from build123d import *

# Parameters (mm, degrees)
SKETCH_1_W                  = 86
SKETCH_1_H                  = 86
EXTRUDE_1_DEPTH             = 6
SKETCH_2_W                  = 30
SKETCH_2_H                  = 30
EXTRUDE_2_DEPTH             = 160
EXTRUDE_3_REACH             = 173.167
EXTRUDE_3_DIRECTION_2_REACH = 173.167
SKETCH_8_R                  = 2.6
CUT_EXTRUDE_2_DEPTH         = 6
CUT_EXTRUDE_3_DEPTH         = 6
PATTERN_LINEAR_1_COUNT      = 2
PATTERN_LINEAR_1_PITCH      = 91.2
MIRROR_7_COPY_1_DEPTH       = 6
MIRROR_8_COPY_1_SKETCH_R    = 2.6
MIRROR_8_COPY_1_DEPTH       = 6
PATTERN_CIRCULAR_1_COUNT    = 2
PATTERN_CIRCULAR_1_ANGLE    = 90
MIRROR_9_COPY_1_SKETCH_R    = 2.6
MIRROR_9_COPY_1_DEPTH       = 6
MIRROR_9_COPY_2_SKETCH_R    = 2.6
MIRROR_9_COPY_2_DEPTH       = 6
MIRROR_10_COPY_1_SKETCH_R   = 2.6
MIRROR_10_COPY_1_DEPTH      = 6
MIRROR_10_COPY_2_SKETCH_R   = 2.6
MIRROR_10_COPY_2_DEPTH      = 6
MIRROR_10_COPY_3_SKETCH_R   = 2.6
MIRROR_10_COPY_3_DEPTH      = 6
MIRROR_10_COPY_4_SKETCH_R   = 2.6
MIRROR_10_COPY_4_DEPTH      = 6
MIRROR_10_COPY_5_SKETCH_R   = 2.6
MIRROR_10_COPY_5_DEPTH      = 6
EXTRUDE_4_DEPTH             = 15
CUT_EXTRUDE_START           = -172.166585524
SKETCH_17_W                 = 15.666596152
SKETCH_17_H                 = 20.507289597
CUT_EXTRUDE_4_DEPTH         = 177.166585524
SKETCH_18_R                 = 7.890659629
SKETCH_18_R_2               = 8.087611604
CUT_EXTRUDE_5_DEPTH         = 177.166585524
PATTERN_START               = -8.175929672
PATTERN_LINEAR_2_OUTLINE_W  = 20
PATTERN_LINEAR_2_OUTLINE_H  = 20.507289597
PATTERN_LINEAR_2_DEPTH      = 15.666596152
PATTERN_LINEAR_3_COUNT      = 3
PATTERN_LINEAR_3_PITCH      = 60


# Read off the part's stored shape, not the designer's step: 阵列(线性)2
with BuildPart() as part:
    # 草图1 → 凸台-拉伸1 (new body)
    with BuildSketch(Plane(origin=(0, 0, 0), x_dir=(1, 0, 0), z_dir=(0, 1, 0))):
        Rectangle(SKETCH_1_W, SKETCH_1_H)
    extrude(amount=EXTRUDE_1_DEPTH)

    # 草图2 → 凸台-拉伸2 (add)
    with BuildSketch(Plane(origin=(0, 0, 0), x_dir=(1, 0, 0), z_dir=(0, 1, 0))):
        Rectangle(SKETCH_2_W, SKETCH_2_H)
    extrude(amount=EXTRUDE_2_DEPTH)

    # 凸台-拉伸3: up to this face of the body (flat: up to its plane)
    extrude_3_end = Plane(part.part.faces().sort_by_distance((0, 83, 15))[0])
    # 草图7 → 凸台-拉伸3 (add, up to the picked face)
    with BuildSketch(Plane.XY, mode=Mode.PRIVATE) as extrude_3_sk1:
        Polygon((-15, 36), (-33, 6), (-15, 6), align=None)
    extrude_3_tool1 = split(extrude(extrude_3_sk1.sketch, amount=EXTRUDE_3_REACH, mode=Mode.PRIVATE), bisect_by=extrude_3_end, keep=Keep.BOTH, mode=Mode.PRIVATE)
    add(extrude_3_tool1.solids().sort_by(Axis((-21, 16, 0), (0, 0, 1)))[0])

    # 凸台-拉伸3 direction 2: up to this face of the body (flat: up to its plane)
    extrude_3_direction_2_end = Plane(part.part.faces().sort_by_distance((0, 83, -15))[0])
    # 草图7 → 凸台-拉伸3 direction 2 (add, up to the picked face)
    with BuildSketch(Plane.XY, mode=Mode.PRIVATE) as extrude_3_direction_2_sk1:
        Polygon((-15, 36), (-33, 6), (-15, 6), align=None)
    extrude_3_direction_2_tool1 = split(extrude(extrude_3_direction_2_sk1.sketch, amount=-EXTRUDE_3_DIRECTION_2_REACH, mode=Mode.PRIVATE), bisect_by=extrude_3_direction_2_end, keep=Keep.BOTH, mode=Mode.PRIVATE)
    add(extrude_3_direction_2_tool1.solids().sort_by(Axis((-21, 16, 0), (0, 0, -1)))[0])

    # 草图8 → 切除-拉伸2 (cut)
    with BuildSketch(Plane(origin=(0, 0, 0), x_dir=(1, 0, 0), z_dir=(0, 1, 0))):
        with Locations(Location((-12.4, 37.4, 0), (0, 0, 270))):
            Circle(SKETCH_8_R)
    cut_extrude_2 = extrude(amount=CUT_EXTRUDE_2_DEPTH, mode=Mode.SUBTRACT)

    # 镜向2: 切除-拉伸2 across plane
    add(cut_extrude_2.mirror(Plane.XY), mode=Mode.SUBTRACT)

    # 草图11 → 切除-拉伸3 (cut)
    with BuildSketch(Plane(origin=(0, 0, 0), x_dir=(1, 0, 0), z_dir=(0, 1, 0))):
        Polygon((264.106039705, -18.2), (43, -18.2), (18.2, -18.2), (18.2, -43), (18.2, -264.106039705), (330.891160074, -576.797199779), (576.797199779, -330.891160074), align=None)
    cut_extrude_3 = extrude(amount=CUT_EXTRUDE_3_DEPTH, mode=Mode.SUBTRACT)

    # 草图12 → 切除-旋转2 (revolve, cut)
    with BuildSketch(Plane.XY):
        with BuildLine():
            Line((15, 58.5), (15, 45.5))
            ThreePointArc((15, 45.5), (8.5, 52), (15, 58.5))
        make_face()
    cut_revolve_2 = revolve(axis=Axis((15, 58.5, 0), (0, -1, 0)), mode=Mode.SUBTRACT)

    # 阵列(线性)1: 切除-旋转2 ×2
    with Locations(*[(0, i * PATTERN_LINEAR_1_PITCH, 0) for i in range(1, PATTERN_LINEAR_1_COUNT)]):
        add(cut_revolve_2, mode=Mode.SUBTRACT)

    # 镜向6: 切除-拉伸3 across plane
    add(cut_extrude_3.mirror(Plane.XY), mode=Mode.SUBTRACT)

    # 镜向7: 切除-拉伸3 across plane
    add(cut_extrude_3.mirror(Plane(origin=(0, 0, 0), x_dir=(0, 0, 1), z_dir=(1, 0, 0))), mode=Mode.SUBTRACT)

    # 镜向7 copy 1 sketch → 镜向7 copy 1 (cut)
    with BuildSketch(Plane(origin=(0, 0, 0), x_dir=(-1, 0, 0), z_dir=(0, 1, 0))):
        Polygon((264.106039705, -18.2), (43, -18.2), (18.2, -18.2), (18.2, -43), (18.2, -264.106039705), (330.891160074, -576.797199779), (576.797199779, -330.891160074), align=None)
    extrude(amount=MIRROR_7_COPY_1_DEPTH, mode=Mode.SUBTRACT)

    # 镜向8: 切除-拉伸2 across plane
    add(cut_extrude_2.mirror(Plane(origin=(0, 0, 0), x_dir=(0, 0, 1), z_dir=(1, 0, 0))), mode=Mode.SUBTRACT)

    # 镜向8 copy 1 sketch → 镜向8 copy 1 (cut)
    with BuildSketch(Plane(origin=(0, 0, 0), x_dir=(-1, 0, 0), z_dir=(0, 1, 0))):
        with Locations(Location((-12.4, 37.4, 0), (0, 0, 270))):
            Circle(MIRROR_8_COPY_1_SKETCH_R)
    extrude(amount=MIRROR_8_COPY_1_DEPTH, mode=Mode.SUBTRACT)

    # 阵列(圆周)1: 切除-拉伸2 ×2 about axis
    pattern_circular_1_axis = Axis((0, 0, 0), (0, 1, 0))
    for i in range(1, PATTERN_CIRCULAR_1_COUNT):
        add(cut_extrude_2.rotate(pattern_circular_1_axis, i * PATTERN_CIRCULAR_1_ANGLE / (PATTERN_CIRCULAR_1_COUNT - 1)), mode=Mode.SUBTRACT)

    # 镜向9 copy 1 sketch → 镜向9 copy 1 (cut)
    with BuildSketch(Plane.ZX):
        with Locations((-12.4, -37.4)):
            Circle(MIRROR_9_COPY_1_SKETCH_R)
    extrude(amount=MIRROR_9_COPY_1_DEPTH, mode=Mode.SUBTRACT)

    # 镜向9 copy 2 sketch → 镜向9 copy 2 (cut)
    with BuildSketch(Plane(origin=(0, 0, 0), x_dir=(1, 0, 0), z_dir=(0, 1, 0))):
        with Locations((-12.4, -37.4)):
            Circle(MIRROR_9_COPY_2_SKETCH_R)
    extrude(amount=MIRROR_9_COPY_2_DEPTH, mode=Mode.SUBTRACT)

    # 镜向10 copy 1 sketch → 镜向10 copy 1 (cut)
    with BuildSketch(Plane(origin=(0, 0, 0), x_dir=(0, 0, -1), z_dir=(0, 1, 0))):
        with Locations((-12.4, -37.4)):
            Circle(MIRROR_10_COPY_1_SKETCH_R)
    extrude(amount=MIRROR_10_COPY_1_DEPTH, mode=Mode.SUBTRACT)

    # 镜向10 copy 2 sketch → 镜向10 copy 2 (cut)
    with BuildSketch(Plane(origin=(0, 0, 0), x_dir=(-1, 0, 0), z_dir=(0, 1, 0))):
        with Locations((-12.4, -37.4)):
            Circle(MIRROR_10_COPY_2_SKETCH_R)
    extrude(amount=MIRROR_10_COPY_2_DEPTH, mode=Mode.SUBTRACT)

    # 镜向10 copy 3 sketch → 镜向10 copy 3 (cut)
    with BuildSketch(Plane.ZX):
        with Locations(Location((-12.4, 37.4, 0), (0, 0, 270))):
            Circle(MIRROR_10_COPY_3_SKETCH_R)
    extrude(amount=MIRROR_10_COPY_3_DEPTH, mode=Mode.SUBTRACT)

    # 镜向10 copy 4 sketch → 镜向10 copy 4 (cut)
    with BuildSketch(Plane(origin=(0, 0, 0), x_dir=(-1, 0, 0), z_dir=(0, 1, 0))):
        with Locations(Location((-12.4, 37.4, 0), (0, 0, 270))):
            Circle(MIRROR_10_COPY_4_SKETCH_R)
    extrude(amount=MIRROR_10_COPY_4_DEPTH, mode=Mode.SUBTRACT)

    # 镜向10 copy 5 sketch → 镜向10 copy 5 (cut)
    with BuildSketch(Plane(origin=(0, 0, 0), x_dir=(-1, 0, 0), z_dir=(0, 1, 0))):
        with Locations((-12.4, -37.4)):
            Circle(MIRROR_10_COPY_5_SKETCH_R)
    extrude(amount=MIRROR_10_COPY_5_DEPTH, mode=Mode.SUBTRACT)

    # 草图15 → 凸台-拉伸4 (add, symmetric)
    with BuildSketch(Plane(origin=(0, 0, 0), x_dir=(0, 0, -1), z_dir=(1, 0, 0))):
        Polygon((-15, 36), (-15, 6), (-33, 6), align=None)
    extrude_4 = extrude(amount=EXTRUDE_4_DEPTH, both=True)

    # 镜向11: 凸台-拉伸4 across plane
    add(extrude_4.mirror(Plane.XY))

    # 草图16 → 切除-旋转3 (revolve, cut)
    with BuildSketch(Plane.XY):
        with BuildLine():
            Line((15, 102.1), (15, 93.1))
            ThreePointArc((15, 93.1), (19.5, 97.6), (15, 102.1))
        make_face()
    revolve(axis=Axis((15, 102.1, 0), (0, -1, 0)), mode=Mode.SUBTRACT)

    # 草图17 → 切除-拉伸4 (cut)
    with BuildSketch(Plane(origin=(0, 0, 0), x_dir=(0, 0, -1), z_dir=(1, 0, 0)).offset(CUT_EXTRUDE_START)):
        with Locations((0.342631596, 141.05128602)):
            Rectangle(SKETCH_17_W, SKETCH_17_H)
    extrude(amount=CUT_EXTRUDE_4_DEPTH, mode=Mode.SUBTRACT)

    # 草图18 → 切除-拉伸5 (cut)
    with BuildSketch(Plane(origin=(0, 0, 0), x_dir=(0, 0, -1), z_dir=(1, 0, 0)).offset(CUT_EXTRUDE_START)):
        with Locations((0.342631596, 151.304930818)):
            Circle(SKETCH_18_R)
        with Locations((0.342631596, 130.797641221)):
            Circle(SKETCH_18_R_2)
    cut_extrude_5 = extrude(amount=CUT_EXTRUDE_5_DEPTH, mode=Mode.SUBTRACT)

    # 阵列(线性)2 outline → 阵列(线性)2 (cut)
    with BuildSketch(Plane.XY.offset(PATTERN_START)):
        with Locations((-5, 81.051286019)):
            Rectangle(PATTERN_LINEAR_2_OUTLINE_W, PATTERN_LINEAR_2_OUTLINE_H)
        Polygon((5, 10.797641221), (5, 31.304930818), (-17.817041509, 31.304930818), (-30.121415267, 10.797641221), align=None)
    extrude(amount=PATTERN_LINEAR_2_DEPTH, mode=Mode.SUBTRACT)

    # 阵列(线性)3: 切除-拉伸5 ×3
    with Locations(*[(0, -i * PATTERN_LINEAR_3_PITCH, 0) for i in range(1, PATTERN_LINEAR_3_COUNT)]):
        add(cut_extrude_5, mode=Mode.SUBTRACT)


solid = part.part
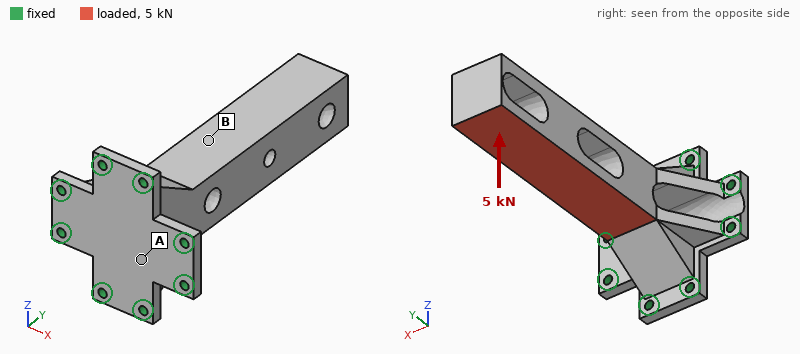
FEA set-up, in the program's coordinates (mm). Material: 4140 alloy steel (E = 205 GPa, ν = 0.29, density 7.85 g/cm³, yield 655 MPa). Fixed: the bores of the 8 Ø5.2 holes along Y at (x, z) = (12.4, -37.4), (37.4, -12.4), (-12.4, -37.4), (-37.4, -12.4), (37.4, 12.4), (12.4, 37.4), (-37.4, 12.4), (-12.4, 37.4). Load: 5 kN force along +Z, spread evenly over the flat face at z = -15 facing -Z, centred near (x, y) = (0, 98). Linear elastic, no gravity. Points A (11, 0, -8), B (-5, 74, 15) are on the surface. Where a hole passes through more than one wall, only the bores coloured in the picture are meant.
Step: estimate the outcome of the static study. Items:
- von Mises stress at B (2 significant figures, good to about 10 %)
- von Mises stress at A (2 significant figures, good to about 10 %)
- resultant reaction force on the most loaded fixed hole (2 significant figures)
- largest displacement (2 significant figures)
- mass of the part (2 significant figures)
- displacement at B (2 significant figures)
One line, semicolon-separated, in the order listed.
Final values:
47 MPa; 18 MPa; 3.7 kN; 0.21 mm; 1.2 kg; 0.057 mm
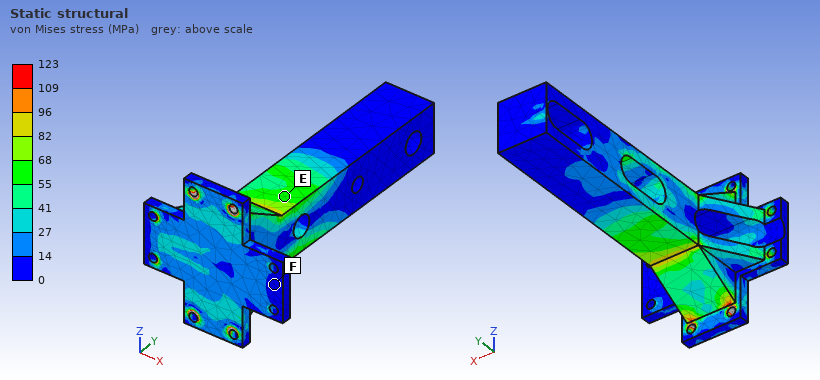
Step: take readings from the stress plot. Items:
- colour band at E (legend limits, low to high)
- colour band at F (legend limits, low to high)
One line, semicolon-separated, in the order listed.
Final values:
55 to 68 MPa; 0 to 14 MPa
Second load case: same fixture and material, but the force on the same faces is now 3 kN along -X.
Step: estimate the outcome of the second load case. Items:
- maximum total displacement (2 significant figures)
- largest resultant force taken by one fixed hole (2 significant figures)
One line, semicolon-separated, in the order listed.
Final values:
0.19 mm; 3.2 kN
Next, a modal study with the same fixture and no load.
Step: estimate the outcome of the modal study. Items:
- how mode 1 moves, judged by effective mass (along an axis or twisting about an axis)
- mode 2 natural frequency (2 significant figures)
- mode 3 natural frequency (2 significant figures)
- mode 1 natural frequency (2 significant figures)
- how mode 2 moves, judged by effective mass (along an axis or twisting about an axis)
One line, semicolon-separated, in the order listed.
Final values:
along X; 1200 Hz; 4100 Hz; 990 Hz; along Z
